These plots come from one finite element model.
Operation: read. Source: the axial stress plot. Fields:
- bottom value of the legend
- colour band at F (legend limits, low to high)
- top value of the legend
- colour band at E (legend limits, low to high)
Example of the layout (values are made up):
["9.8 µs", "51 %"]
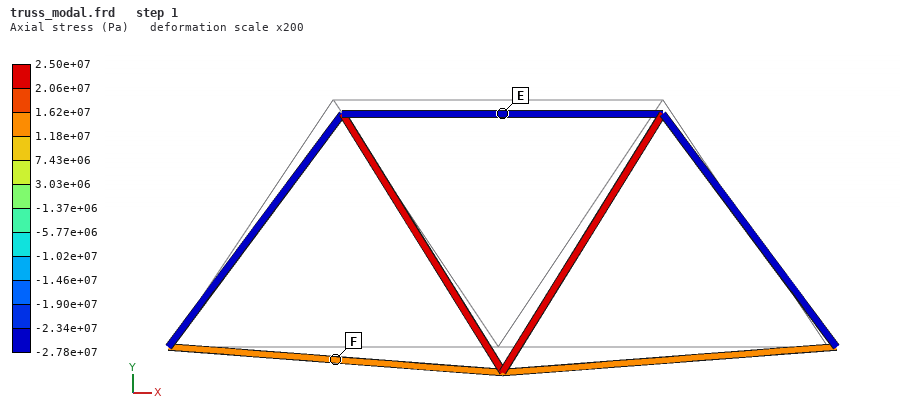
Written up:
["-2.78e+07 Pa", "1.18e+07 to 1.62e+07 Pa", "2.50e+07 Pa", "-2.78e+07 to -2.34e+07 Pa"]
